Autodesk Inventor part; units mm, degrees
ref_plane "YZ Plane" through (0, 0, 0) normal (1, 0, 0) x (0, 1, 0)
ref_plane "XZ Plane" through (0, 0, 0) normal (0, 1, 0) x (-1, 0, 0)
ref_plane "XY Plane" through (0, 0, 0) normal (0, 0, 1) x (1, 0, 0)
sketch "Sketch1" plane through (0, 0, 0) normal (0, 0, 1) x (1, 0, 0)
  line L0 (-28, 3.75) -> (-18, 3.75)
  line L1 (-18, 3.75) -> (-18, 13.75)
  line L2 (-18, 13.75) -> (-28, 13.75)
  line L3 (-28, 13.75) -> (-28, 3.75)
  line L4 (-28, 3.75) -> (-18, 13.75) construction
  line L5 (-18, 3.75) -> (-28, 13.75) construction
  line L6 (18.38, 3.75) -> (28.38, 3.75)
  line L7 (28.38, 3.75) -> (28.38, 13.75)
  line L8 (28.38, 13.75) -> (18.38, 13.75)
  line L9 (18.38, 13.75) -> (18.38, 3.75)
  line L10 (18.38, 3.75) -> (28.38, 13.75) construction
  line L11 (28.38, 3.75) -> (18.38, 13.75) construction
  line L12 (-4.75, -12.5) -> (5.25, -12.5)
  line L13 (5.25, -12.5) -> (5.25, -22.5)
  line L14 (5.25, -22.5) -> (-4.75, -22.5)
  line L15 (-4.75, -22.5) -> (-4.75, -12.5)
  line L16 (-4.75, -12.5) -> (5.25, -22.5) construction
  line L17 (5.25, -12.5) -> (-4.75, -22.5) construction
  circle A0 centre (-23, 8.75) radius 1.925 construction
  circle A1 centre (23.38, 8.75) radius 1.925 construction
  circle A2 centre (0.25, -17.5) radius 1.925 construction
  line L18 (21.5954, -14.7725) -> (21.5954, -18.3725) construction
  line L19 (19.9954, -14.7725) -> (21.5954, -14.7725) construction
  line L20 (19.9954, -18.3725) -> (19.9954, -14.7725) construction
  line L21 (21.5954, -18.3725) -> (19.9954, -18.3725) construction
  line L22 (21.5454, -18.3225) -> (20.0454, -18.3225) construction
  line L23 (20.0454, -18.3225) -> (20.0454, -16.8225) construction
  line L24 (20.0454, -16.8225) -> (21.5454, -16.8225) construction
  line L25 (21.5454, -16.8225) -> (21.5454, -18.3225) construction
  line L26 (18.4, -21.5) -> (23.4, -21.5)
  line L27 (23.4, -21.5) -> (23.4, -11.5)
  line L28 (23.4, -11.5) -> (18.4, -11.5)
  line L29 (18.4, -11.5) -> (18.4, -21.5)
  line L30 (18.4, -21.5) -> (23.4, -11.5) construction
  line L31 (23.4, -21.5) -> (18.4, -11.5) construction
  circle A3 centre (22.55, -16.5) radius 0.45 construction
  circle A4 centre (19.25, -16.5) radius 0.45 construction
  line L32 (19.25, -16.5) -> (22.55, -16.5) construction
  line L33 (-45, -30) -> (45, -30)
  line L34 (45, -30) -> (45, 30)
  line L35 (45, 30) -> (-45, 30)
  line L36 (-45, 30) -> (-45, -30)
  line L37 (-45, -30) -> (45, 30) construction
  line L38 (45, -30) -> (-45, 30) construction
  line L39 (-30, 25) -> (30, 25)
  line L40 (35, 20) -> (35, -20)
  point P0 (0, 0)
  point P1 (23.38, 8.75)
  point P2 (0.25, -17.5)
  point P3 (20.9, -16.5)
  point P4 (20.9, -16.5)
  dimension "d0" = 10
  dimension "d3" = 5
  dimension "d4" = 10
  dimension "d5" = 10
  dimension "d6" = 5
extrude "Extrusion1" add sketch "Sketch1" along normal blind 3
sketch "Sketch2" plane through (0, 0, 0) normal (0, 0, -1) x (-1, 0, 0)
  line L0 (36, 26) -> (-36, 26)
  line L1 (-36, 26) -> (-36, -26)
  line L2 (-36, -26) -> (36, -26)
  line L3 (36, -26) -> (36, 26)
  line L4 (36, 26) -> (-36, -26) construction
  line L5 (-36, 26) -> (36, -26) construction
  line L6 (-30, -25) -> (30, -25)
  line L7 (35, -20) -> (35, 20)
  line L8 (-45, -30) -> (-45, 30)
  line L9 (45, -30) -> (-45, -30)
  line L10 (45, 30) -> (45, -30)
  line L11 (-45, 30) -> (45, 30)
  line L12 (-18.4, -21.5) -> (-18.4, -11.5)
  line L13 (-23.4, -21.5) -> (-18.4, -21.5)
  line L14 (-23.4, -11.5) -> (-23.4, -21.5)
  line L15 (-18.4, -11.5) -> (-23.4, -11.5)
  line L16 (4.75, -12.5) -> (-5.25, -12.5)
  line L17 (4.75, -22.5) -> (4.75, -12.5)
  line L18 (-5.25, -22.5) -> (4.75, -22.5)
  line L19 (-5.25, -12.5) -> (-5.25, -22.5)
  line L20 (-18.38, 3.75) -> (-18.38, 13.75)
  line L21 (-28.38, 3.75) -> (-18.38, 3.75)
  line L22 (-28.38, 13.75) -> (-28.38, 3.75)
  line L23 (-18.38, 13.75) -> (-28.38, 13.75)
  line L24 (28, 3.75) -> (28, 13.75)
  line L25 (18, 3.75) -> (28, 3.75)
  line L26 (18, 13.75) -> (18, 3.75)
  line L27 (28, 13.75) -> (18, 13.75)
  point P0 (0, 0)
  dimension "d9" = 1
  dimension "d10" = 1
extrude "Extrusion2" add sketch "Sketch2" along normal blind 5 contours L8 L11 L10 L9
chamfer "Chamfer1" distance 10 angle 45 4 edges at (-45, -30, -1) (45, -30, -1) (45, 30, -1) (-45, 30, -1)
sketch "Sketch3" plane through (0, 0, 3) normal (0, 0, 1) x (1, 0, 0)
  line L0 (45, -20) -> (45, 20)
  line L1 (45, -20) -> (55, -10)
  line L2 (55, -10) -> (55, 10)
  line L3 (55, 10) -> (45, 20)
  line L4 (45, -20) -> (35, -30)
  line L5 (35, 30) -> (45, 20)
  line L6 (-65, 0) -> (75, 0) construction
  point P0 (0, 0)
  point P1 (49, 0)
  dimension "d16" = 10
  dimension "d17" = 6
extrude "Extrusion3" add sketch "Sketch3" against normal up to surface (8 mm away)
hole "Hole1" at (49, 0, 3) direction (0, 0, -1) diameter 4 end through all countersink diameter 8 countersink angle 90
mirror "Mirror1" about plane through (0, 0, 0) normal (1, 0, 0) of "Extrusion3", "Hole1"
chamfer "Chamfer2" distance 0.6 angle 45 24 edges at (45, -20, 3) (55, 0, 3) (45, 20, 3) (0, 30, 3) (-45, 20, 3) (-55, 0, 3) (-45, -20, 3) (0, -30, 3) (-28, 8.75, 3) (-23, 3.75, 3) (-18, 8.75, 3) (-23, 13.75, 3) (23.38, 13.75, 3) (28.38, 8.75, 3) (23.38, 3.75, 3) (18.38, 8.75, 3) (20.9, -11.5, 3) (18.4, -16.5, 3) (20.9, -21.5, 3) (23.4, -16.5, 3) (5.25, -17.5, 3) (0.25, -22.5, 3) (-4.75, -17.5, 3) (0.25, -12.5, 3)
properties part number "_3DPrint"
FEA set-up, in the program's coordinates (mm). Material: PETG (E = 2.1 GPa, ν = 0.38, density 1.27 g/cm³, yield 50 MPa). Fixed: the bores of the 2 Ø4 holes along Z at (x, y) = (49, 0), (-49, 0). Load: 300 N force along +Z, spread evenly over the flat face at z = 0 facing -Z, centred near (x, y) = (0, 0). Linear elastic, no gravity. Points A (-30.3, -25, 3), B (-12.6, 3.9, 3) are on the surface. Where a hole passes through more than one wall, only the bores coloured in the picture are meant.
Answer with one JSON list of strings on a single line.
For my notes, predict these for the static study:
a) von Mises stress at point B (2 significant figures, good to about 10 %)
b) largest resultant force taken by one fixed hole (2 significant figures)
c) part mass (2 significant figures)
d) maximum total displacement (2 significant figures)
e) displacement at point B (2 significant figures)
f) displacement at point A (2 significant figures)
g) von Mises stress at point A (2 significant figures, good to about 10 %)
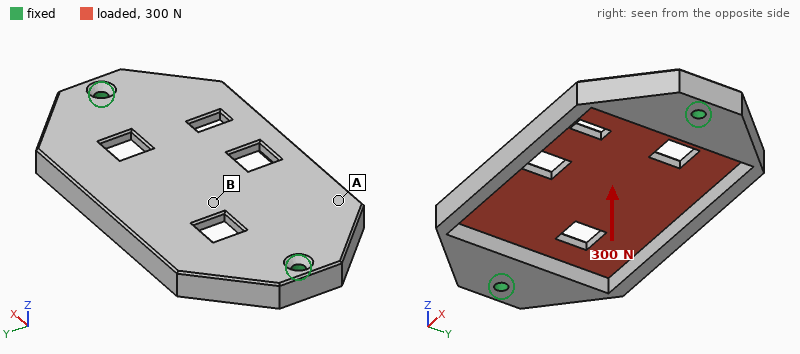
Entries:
["7.6 MPa", "210 N", "33 g", "1.2 mm", "1.0 mm", "0.41 mm", "2.5 MPa"]
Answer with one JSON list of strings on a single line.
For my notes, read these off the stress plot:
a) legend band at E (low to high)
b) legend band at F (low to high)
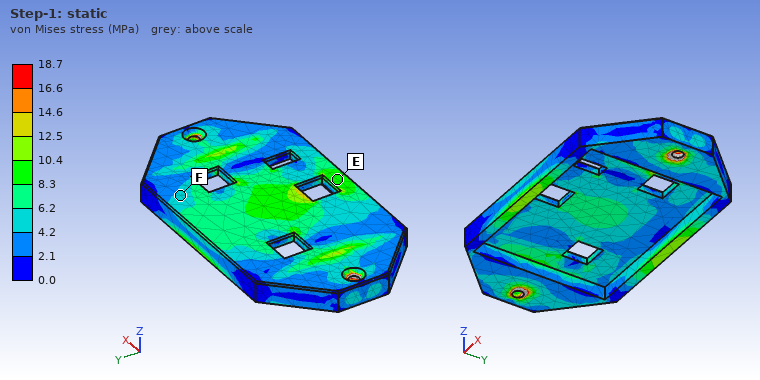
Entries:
["8.3 to 10.4 MPa", "4.2 to 6.2 MPa"]
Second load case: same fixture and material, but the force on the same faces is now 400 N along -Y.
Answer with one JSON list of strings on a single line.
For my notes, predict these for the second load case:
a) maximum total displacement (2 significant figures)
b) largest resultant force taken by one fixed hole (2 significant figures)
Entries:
["0.13 mm", "200 N"]
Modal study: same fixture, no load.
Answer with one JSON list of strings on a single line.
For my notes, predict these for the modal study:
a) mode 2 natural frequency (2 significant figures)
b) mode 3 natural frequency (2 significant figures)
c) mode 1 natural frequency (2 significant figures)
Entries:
["700 Hz", "1400 Hz", "700 Hz"]
